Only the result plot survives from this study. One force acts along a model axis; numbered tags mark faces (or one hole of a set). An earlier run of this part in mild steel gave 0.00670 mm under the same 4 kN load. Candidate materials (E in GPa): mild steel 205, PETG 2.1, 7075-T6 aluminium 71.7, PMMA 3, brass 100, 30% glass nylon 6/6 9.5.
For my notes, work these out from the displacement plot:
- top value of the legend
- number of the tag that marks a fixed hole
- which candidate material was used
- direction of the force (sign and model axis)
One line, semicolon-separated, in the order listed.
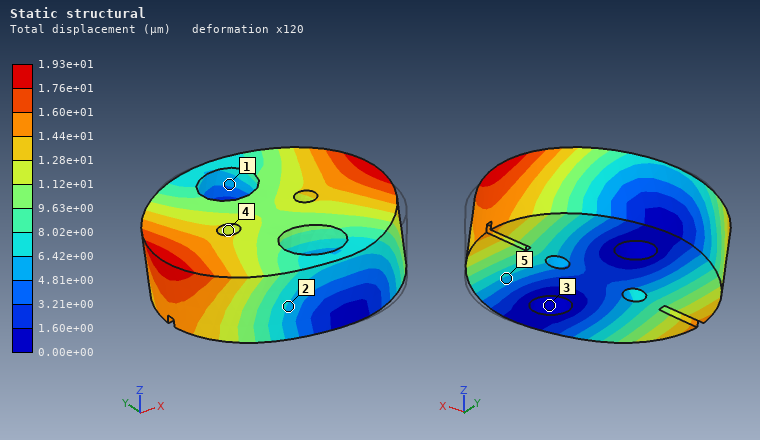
1.93e+01 µm; 3; 7075-T6 aluminium; -X
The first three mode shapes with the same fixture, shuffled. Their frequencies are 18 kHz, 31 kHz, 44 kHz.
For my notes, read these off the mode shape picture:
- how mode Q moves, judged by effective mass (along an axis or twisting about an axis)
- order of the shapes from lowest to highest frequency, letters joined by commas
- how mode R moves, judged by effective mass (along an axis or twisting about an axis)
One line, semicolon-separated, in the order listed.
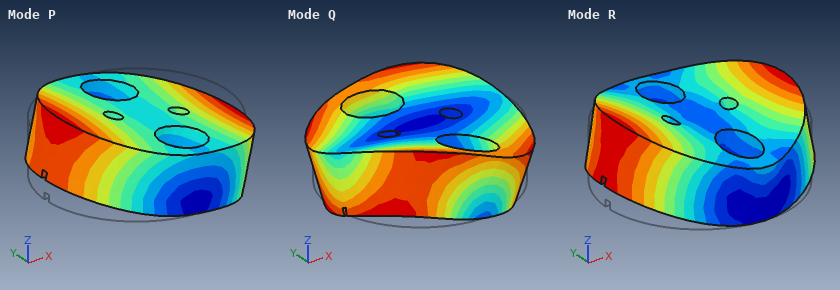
twisting about Z; P, R, Q; along Z
